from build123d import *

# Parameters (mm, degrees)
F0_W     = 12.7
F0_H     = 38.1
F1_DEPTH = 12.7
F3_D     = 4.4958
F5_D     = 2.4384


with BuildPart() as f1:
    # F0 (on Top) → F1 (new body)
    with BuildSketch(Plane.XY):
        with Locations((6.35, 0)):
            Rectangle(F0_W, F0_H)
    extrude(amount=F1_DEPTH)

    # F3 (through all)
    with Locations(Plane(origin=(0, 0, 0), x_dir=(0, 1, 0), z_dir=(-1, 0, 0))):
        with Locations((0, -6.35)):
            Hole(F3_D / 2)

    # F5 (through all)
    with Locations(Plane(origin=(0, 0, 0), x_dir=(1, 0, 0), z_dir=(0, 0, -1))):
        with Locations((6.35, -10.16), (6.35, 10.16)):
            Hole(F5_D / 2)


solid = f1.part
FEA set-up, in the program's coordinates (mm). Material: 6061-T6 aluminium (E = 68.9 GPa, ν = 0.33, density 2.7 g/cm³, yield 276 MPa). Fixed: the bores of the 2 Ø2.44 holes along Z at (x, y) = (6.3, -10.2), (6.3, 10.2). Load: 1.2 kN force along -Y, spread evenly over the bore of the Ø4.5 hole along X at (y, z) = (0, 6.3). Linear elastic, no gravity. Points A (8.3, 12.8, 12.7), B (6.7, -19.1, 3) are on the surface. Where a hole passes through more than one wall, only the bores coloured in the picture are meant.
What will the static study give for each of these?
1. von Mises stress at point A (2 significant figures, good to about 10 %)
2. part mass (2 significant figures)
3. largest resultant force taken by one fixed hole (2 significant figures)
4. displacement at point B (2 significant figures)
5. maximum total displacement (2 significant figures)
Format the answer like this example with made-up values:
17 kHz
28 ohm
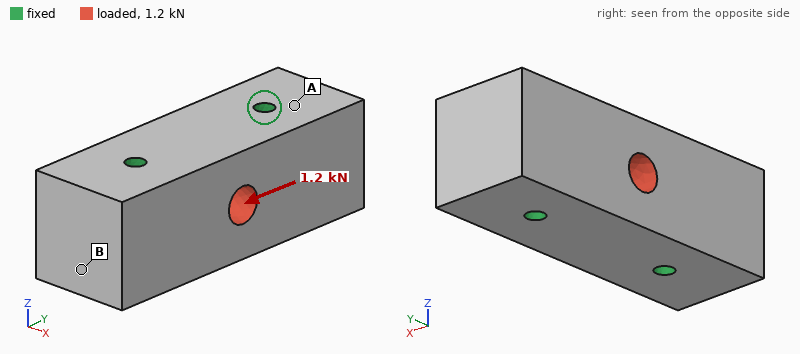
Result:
2.4 MPa
16 g
600 N
0.14 µm
0.82 µm
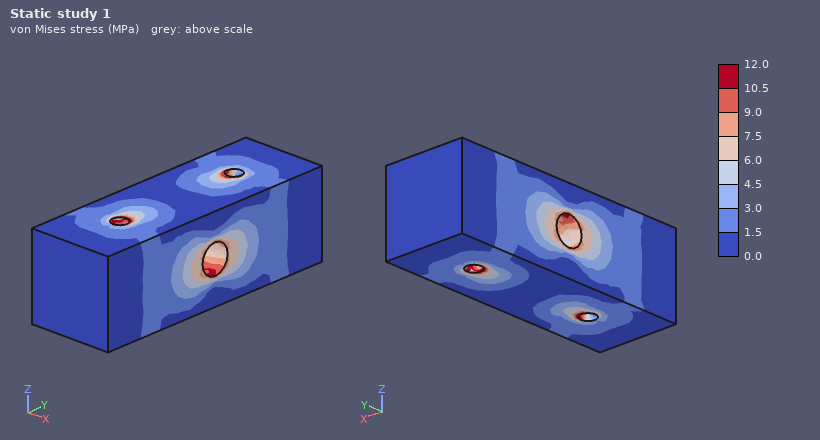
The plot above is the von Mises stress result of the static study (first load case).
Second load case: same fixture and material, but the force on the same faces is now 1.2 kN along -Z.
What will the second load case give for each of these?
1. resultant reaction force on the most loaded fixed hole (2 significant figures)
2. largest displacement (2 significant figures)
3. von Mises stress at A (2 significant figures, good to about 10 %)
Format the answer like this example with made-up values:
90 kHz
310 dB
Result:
600 N
2.3 µm
4.7 MPa
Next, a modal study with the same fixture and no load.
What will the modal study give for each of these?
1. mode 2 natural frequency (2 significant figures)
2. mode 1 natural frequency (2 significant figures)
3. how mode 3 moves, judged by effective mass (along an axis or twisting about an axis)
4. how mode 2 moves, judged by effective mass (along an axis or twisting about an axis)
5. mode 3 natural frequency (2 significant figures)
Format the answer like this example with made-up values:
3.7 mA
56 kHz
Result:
46 kHz
39 kHz
twisting about X
twisting about Z
57 kHz
